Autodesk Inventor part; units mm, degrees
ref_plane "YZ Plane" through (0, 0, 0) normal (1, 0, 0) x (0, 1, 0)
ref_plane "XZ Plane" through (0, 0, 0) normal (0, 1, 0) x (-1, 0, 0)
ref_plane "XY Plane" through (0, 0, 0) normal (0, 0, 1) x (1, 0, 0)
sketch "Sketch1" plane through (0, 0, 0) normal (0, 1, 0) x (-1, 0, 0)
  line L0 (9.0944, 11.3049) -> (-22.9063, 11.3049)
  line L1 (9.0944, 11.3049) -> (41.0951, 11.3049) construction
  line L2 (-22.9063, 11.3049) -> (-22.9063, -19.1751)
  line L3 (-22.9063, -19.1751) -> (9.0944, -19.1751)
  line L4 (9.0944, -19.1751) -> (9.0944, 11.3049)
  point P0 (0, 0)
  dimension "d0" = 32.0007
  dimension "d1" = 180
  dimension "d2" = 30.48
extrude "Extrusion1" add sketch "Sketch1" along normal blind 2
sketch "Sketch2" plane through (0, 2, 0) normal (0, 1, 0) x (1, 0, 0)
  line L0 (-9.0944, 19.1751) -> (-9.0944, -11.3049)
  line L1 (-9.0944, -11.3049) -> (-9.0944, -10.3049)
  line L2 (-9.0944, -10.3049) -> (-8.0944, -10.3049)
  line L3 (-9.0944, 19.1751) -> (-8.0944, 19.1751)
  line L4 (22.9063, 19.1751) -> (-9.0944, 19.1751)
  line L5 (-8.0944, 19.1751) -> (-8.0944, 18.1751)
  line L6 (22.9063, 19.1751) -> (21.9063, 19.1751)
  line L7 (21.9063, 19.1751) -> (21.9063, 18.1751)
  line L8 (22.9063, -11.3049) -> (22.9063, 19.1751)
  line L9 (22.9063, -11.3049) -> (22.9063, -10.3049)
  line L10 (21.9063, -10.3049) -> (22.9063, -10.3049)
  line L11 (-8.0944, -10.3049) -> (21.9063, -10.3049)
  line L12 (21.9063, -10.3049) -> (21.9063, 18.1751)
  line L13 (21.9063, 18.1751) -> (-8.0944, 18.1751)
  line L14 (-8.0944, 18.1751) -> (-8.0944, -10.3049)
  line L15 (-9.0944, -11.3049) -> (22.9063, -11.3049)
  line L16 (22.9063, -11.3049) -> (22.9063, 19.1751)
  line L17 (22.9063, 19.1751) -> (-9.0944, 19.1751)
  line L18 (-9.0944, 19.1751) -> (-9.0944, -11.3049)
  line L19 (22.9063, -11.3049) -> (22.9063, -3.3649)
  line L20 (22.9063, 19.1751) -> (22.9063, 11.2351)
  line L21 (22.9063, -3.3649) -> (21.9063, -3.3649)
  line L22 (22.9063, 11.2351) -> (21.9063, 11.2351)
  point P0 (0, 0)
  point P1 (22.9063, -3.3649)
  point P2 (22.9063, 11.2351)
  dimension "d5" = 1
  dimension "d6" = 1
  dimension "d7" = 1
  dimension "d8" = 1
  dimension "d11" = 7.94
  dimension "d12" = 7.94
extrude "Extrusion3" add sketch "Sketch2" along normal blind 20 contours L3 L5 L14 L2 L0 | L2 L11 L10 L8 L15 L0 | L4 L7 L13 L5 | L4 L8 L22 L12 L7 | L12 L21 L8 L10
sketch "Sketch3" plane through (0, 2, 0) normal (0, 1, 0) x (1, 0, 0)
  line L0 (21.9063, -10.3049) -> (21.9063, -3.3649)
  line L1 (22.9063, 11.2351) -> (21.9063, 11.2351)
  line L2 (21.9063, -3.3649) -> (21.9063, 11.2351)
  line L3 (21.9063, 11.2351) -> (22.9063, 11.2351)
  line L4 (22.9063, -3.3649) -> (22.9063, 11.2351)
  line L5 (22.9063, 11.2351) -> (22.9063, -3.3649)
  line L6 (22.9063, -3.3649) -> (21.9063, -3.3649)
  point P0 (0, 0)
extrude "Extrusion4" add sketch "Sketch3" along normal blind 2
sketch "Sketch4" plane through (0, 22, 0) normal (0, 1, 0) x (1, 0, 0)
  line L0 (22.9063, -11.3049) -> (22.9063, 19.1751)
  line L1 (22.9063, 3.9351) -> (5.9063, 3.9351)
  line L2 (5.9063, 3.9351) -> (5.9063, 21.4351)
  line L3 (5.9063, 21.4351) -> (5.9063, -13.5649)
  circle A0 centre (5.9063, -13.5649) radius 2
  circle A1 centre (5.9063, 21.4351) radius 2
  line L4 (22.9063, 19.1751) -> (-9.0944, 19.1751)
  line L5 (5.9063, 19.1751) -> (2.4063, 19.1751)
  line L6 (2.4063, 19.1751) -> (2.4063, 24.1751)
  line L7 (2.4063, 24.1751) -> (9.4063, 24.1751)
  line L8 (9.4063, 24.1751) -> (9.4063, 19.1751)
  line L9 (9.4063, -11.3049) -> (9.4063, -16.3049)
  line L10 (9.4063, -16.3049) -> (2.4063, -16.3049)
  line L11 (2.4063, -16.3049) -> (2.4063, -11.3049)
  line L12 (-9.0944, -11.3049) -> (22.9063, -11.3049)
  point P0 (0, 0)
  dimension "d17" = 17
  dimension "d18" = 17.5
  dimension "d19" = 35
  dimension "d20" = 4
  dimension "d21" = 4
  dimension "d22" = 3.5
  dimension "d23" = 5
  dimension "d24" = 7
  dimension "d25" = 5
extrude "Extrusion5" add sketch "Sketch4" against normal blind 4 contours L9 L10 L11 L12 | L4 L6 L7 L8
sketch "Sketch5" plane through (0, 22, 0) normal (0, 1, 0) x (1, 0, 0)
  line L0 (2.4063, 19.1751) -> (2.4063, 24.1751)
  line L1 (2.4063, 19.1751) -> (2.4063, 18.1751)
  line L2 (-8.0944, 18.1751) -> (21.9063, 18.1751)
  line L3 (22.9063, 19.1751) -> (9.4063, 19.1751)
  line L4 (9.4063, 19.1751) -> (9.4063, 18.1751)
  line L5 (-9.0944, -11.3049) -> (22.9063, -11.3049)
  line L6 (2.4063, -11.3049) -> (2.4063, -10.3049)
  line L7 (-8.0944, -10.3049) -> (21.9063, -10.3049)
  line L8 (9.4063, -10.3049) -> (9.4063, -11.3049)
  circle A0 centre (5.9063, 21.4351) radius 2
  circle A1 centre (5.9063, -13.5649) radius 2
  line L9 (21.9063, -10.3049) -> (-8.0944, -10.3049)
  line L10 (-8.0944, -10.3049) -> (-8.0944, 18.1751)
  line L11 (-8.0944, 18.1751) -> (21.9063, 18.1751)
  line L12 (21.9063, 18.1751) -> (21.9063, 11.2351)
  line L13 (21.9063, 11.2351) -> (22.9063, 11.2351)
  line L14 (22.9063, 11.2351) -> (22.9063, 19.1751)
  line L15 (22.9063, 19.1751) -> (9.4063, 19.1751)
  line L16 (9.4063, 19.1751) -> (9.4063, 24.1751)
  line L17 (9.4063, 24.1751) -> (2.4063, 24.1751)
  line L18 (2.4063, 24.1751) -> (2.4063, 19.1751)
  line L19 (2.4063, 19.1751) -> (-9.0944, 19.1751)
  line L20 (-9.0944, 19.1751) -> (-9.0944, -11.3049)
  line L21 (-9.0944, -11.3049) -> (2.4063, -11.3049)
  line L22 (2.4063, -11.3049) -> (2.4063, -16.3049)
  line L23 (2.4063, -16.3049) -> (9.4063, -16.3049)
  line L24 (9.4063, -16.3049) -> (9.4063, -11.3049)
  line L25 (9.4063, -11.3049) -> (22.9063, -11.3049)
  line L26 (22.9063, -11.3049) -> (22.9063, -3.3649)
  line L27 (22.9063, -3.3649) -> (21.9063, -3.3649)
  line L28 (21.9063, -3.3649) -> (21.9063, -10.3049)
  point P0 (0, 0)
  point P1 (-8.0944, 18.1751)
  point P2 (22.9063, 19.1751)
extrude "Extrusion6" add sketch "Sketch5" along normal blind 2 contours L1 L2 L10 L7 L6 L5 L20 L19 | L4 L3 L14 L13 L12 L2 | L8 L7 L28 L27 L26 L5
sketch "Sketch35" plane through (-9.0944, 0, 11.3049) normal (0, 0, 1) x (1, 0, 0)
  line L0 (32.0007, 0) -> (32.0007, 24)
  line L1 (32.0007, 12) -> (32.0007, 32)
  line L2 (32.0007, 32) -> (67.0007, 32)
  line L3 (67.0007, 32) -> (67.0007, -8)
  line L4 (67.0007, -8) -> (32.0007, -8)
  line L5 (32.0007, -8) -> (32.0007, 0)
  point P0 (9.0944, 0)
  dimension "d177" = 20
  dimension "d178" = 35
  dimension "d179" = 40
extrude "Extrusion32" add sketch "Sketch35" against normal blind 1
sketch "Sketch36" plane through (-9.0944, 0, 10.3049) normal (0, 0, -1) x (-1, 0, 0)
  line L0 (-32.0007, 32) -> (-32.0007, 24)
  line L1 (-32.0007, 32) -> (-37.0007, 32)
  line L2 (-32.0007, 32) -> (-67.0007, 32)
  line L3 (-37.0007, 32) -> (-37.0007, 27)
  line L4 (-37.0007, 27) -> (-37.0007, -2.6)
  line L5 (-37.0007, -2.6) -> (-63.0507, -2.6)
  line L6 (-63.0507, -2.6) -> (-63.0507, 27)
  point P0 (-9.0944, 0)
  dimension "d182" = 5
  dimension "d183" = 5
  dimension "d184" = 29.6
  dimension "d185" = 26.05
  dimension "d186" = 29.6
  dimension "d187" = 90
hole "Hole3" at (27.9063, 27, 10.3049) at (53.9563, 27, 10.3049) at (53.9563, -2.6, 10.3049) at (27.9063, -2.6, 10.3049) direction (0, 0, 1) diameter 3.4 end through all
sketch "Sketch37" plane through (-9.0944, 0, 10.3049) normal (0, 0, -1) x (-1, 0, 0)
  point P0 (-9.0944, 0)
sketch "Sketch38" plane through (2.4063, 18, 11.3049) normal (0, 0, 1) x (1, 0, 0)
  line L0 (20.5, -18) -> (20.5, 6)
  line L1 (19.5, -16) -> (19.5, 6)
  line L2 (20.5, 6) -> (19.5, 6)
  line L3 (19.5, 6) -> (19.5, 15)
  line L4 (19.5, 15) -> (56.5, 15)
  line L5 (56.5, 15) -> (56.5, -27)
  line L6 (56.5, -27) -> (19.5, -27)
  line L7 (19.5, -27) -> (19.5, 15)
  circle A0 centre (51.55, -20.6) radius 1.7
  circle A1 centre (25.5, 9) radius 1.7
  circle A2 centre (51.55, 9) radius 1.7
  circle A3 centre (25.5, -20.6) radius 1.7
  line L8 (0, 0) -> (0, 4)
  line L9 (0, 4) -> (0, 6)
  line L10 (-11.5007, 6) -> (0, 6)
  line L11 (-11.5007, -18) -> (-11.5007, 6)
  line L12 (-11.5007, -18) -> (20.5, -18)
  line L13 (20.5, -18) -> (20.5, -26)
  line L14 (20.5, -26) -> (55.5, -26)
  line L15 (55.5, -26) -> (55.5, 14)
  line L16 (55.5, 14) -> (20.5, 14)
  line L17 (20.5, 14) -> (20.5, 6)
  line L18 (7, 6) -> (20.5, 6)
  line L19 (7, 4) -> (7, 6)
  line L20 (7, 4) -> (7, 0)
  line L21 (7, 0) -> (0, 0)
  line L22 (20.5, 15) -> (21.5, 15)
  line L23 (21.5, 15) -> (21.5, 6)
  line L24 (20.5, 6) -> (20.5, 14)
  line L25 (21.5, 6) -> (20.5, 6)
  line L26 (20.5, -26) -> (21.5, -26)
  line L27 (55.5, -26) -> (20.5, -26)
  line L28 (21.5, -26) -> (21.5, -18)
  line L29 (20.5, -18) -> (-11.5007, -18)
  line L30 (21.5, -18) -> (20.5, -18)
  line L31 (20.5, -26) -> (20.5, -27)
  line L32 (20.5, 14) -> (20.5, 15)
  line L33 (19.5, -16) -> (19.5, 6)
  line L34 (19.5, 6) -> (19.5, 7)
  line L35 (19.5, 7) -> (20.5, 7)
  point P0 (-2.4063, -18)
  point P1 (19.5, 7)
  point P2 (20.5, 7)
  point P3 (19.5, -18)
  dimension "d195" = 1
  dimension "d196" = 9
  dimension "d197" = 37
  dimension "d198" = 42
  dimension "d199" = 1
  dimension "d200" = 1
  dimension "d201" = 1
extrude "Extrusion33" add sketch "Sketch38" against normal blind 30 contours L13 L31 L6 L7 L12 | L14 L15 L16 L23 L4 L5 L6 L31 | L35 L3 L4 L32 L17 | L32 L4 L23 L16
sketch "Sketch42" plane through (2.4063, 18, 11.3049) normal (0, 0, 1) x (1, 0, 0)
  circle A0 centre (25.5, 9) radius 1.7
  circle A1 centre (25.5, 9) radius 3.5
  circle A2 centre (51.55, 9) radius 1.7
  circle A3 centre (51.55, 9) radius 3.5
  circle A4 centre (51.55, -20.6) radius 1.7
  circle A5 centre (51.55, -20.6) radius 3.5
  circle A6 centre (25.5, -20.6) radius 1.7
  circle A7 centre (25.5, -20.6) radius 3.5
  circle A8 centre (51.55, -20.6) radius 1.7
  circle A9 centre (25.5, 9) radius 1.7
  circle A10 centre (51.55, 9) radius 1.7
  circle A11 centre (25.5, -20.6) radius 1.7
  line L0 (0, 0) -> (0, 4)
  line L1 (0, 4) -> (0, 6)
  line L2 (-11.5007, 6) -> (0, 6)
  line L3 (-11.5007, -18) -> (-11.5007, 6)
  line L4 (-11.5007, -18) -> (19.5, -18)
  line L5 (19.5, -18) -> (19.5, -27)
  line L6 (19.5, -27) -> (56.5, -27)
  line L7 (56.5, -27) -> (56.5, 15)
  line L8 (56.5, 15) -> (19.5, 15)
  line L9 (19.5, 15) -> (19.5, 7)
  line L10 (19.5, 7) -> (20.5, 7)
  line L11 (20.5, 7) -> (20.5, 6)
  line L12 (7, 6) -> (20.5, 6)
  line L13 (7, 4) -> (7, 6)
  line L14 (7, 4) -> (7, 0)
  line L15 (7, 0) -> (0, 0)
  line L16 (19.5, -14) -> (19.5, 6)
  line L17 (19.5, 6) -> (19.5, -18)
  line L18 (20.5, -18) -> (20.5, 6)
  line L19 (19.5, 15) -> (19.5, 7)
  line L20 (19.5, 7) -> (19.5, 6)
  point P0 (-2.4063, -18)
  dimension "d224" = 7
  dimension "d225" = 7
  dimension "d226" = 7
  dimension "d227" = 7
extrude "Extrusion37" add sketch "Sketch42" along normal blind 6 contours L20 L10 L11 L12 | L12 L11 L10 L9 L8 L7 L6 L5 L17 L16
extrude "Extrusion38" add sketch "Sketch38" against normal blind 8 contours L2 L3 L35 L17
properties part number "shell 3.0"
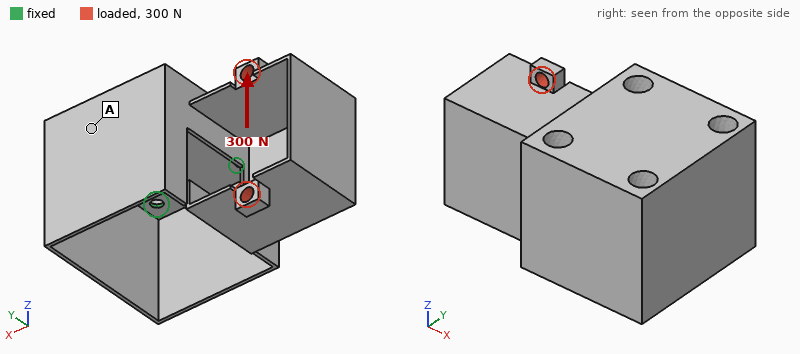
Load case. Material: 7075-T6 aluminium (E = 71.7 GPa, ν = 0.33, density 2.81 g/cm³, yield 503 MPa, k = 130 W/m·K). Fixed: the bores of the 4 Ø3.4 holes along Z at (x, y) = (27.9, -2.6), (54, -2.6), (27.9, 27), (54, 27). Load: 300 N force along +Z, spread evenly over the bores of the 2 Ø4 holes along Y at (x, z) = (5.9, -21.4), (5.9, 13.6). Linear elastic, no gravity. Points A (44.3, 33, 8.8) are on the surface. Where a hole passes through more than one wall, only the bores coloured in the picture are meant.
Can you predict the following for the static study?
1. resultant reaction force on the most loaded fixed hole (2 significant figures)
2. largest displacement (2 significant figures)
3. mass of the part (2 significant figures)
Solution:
330 N
1.1 mm
51 g
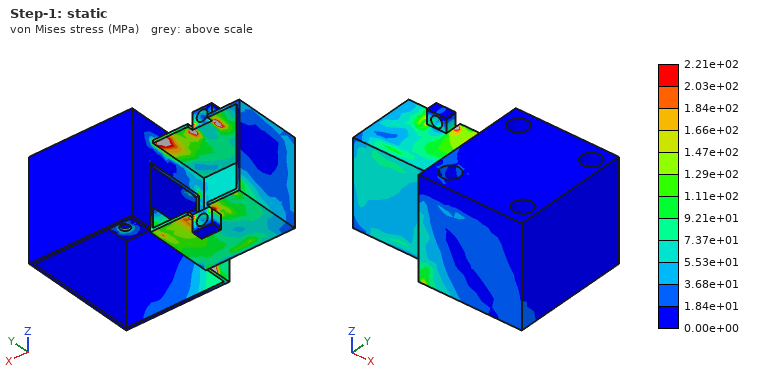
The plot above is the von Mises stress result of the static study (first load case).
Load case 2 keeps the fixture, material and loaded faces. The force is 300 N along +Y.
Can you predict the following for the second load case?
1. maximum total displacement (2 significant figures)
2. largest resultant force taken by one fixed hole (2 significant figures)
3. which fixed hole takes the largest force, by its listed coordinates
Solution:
0.87 mm
390 N
(27.9, -2.6)
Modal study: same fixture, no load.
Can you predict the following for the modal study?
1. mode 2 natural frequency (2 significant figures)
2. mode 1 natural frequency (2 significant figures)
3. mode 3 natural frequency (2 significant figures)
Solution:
1300 Hz
930 Hz
2600 Hz
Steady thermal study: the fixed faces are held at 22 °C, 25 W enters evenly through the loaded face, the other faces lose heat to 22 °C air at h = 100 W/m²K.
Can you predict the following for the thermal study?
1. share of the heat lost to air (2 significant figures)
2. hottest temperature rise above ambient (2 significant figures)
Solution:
76 %
78 K
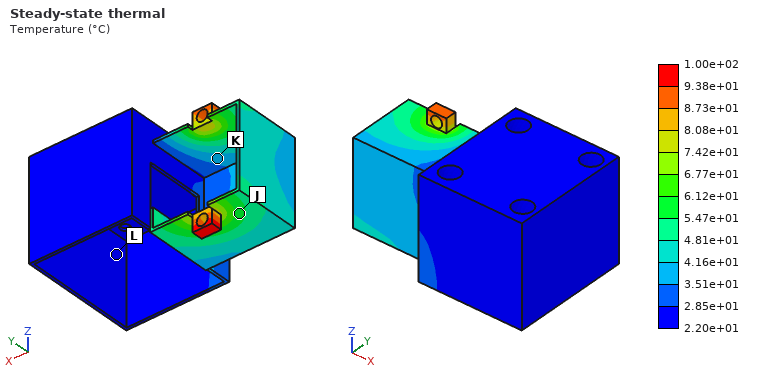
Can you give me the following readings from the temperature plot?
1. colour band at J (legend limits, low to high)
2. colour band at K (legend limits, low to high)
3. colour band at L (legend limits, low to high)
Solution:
5.47e+01 to 6.12e+01 °C
3.51e+01 to 4.16e+01 °C
2.20e+01 to 2.85e+01 °C
